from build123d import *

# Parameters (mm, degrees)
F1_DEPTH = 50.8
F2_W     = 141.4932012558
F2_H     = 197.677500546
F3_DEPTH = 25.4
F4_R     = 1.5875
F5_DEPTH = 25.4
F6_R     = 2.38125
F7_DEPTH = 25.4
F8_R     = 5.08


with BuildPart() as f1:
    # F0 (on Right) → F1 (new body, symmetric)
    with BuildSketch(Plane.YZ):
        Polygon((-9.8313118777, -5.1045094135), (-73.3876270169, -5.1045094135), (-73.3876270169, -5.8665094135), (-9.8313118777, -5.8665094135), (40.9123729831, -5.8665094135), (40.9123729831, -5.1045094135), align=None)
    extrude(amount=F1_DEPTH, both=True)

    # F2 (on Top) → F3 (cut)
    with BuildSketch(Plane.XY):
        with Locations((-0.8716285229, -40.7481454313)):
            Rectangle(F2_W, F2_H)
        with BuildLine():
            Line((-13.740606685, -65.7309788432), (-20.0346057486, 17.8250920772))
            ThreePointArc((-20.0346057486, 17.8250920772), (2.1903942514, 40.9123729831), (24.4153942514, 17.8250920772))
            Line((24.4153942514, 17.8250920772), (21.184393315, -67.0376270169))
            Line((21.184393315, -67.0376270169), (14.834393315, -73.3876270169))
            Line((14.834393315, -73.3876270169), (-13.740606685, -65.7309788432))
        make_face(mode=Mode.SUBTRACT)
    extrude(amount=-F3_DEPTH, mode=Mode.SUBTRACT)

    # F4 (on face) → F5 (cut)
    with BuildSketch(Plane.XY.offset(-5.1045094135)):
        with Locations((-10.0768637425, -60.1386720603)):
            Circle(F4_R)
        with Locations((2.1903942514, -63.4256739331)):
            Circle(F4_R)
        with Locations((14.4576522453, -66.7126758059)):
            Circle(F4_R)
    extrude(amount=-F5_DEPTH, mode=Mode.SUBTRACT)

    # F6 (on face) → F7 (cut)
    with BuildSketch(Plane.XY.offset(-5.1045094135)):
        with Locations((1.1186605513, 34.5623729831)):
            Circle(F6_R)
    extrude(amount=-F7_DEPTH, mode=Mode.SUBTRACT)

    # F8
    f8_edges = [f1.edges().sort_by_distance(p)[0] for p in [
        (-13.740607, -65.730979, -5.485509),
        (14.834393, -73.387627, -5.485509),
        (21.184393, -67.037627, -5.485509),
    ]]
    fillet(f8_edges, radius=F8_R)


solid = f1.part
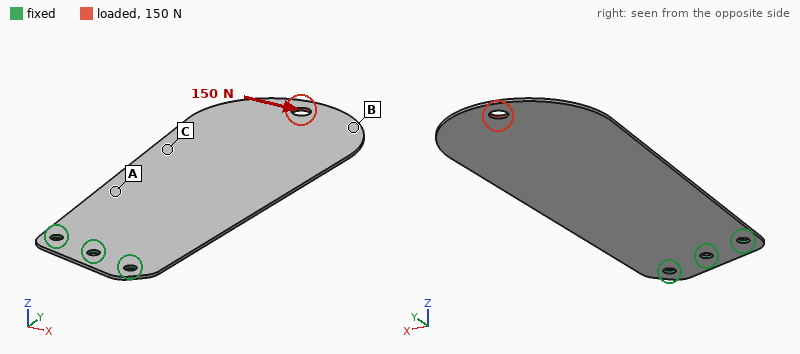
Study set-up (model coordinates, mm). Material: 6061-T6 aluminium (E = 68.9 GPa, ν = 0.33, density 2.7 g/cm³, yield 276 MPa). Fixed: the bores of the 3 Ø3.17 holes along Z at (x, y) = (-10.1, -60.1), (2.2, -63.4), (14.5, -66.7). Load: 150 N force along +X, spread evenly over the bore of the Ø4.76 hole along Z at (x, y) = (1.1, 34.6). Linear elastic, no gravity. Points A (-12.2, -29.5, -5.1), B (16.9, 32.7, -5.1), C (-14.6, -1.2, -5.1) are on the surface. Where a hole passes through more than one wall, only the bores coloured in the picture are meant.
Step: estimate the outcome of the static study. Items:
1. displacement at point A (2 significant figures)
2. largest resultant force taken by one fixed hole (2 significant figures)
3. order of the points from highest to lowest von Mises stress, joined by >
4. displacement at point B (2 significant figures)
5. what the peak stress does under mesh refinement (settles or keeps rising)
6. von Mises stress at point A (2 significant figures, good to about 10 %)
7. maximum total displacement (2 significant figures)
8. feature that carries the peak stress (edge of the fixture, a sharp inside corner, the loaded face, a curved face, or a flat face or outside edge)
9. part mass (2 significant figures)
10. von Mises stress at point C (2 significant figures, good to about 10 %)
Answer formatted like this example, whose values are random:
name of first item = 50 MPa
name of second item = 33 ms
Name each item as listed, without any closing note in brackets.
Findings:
displacement at point A = 0.056 mm
largest resultant force taken by one fixed hole = 580 N
order of the points from highest to lowest von Mises stress, joined by > = A > C > B
displacement at point B = 0.23 mm
what the peak stress does under mesh refinement = keeps rising
von Mises stress at point A = 39 MPa
maximum total displacement = 0.25 mm
feature that carries the peak stress = edge of the fixture
part mass = 8.7 g
von Mises stress at point C = 19 MPa
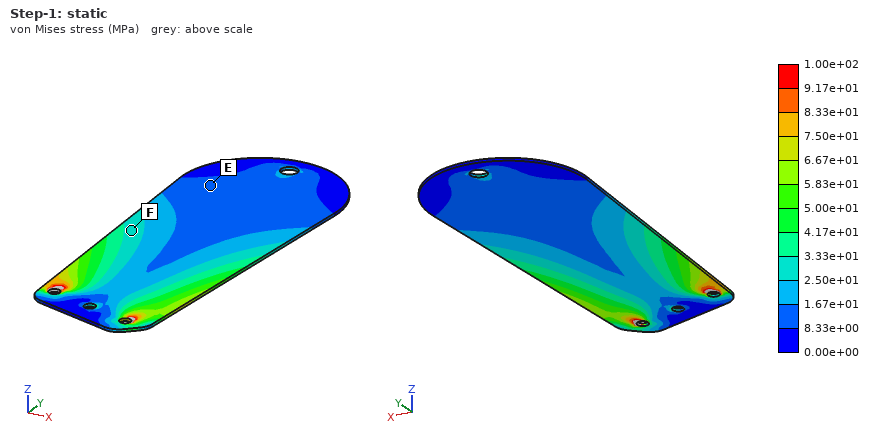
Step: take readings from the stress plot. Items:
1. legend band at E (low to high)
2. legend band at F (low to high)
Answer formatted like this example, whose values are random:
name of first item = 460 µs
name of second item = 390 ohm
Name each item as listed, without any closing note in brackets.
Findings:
legend band at E = 8.33e+00 to 1.67e+01 MPa
legend band at F = 2.50e+01 to 3.33e+01 MPa
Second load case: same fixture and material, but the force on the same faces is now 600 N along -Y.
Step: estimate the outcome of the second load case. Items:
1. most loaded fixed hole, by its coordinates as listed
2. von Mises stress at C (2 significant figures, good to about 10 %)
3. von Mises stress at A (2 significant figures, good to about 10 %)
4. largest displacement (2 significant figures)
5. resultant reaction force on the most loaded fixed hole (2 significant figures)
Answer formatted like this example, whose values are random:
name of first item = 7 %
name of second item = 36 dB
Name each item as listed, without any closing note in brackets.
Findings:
most loaded fixed hole, by its coordinates as listed = (-10.1, -60.1)
von Mises stress at C = 21 MPa
von Mises stress at A = 25 MPa
largest displacement = 42 µm
resultant reaction force on the most loaded fixed hole = 230 N
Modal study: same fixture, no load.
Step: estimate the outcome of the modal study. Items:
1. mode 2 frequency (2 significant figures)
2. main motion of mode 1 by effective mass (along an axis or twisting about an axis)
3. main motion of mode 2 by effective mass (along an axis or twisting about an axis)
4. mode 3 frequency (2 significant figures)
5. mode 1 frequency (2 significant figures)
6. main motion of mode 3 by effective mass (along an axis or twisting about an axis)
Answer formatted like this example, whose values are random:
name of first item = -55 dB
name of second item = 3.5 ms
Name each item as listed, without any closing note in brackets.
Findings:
mode 2 frequency = 310 Hz
main motion of mode 1 by effective mass = along Z
main motion of mode 2 by effective mass = twisting about Y
mode 3 frequency = 400 Hz
mode 1 frequency = 61 Hz
main motion of mode 3 by effective mass = along Z
